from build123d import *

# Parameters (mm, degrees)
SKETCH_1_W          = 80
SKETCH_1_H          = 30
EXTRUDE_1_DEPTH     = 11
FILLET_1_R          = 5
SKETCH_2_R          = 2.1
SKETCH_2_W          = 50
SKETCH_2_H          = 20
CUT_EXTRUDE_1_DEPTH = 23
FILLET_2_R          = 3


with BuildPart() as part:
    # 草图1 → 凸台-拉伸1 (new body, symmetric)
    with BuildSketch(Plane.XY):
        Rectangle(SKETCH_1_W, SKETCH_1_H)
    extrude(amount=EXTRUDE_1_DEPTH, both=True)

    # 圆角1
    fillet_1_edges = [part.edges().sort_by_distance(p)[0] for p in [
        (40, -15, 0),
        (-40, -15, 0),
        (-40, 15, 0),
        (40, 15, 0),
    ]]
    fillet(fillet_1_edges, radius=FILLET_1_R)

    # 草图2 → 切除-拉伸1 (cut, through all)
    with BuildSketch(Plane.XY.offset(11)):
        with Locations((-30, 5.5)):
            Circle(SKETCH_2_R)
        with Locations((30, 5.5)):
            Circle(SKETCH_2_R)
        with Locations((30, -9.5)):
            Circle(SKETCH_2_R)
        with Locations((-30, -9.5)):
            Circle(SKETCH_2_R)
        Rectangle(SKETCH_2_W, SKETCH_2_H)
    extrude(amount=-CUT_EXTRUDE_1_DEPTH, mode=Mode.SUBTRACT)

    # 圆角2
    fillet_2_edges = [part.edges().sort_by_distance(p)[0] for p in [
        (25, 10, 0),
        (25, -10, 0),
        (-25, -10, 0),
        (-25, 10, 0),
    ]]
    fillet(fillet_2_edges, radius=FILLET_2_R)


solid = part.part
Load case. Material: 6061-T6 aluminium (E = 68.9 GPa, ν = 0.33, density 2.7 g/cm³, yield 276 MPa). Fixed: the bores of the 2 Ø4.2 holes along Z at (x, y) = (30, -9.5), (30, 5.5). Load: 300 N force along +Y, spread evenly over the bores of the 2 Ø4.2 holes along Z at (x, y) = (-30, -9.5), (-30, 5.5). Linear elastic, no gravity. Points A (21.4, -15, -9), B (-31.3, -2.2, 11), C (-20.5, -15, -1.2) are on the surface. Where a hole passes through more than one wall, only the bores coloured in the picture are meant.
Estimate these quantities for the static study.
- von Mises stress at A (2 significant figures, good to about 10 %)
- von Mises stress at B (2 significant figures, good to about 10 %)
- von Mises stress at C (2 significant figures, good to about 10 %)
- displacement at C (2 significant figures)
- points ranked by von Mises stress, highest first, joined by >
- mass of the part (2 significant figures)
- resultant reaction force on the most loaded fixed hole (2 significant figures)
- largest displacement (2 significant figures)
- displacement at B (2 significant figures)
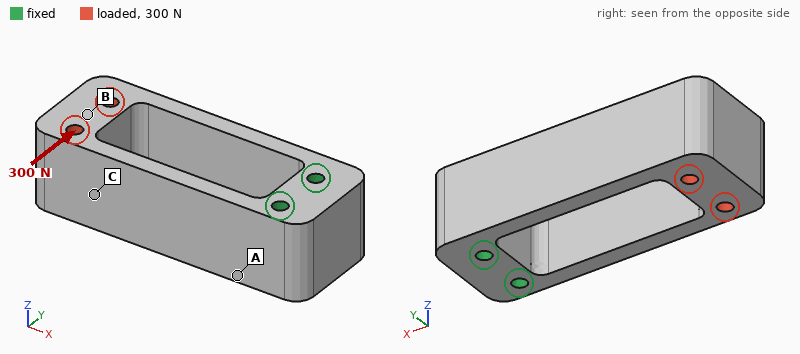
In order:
38 MPa
4.8 MPa
27 MPa
0.12 mm
A > C > B
79 g
840 N
0.13 mm
0.13 mm
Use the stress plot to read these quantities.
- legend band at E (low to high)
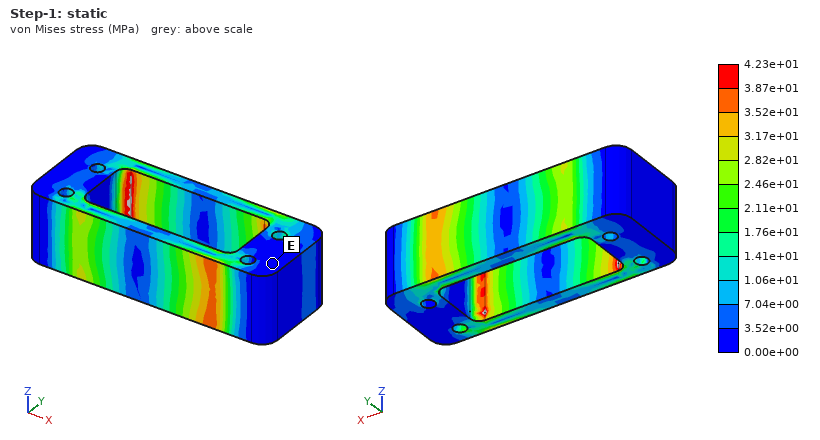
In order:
0.00e+00 to 3.52e+00 MPa
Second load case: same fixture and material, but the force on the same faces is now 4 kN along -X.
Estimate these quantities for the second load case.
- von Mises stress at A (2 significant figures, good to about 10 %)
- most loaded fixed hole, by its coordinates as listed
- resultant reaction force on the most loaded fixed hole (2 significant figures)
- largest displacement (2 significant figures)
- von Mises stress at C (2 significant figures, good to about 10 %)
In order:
20 MPa
(30, -9.5)
2.1 kN
20 µm
17 MPa
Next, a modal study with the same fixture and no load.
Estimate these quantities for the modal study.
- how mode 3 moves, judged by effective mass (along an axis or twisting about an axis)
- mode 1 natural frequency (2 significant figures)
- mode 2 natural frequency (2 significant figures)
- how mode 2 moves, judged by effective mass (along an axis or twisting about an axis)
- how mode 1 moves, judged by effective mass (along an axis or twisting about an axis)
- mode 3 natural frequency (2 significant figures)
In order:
twisting about X
1300 Hz
2300 Hz
along Z
along Y
4700 Hz
